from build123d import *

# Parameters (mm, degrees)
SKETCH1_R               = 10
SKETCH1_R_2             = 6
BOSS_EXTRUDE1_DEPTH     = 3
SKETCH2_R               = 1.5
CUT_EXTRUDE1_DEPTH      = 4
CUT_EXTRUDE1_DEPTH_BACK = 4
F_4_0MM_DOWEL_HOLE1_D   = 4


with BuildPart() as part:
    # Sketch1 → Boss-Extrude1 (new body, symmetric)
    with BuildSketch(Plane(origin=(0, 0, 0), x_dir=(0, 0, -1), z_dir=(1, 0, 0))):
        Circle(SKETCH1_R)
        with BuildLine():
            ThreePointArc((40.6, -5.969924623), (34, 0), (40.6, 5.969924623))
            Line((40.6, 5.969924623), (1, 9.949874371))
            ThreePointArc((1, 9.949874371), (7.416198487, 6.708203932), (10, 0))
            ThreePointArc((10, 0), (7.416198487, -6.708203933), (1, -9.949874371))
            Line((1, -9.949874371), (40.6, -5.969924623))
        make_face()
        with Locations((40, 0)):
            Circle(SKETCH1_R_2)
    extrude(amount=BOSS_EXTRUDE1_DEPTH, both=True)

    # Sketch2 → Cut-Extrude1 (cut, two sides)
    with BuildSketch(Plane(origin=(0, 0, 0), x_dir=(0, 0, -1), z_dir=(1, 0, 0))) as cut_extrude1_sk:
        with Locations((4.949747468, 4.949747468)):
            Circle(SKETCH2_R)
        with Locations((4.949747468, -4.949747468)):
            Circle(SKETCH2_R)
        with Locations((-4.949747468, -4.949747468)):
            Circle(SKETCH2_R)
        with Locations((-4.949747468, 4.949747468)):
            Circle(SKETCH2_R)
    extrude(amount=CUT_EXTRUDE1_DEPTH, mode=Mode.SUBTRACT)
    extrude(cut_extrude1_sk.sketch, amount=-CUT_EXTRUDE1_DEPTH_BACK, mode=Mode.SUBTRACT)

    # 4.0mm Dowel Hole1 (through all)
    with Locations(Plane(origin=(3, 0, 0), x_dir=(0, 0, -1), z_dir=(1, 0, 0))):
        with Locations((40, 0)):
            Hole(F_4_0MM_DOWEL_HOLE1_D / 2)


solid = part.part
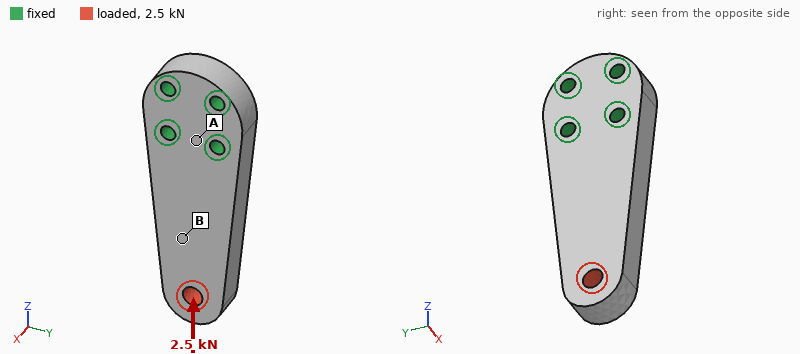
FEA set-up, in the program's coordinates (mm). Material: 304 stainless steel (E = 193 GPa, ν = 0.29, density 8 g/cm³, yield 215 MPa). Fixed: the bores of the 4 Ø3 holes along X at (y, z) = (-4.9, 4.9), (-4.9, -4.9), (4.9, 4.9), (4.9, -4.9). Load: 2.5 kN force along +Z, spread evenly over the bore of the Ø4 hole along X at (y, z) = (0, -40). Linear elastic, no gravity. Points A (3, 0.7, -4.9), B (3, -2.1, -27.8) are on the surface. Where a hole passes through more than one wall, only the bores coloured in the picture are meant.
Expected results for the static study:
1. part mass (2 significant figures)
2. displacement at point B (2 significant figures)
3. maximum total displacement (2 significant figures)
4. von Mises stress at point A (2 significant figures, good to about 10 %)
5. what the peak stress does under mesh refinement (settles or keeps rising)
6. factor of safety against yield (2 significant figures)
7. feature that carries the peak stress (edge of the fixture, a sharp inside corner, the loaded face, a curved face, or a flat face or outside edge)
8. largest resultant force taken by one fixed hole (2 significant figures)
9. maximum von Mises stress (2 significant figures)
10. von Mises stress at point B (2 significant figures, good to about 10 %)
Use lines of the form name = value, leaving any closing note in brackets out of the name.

part mass = 39 g
displacement at point B = 3.0 µm
maximum total displacement = 6.2 µm
von Mises stress at point A = 10 MPa
what the peak stress does under mesh refinement = settles
factor of safety against yield = 2.6
feature that carries the peak stress = the loaded face
largest resultant force taken by one fixed hole = 1.1 kN
maximum von Mises stress = 82 MPa
von Mises stress at point B = 29 MPa
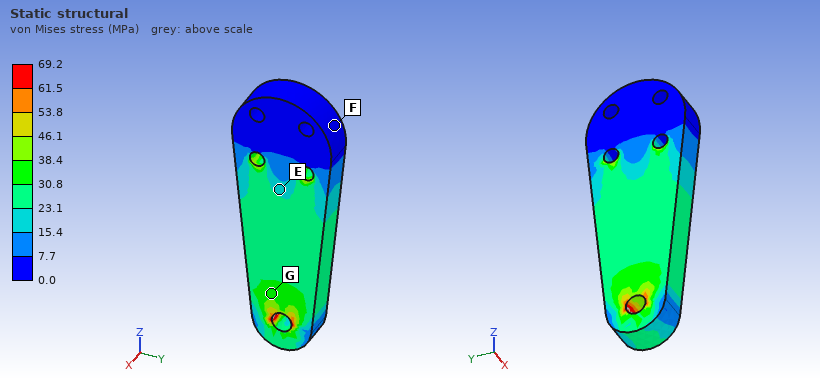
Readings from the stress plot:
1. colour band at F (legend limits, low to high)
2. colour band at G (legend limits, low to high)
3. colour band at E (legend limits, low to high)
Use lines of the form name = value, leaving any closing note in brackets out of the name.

colour band at F = 0.0 to 7.7 MPa
colour band at G = 30.8 to 38.4 MPa
colour band at E = 15.4 to 23.1 MPa
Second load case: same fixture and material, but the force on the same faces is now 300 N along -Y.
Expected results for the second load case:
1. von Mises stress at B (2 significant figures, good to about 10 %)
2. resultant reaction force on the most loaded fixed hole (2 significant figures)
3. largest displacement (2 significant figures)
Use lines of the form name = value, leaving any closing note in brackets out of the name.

von Mises stress at B = 8.6 MPa
resultant reaction force on the most loaded fixed hole = 780 N
largest displacement = 14 µm
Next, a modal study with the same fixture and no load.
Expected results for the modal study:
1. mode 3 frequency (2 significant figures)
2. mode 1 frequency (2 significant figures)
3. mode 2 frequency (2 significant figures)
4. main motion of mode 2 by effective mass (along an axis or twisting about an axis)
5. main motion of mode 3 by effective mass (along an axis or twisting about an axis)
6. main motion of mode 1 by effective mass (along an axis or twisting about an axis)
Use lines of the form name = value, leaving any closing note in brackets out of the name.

mode 3 frequency = 17 kHz
mode 1 frequency = 3600 Hz
mode 2 frequency = 9200 Hz
main motion of mode 2 by effective mass = along Y
main motion of mode 3 by effective mass = twisting about Z
main motion of mode 1 by effective mass = along X
